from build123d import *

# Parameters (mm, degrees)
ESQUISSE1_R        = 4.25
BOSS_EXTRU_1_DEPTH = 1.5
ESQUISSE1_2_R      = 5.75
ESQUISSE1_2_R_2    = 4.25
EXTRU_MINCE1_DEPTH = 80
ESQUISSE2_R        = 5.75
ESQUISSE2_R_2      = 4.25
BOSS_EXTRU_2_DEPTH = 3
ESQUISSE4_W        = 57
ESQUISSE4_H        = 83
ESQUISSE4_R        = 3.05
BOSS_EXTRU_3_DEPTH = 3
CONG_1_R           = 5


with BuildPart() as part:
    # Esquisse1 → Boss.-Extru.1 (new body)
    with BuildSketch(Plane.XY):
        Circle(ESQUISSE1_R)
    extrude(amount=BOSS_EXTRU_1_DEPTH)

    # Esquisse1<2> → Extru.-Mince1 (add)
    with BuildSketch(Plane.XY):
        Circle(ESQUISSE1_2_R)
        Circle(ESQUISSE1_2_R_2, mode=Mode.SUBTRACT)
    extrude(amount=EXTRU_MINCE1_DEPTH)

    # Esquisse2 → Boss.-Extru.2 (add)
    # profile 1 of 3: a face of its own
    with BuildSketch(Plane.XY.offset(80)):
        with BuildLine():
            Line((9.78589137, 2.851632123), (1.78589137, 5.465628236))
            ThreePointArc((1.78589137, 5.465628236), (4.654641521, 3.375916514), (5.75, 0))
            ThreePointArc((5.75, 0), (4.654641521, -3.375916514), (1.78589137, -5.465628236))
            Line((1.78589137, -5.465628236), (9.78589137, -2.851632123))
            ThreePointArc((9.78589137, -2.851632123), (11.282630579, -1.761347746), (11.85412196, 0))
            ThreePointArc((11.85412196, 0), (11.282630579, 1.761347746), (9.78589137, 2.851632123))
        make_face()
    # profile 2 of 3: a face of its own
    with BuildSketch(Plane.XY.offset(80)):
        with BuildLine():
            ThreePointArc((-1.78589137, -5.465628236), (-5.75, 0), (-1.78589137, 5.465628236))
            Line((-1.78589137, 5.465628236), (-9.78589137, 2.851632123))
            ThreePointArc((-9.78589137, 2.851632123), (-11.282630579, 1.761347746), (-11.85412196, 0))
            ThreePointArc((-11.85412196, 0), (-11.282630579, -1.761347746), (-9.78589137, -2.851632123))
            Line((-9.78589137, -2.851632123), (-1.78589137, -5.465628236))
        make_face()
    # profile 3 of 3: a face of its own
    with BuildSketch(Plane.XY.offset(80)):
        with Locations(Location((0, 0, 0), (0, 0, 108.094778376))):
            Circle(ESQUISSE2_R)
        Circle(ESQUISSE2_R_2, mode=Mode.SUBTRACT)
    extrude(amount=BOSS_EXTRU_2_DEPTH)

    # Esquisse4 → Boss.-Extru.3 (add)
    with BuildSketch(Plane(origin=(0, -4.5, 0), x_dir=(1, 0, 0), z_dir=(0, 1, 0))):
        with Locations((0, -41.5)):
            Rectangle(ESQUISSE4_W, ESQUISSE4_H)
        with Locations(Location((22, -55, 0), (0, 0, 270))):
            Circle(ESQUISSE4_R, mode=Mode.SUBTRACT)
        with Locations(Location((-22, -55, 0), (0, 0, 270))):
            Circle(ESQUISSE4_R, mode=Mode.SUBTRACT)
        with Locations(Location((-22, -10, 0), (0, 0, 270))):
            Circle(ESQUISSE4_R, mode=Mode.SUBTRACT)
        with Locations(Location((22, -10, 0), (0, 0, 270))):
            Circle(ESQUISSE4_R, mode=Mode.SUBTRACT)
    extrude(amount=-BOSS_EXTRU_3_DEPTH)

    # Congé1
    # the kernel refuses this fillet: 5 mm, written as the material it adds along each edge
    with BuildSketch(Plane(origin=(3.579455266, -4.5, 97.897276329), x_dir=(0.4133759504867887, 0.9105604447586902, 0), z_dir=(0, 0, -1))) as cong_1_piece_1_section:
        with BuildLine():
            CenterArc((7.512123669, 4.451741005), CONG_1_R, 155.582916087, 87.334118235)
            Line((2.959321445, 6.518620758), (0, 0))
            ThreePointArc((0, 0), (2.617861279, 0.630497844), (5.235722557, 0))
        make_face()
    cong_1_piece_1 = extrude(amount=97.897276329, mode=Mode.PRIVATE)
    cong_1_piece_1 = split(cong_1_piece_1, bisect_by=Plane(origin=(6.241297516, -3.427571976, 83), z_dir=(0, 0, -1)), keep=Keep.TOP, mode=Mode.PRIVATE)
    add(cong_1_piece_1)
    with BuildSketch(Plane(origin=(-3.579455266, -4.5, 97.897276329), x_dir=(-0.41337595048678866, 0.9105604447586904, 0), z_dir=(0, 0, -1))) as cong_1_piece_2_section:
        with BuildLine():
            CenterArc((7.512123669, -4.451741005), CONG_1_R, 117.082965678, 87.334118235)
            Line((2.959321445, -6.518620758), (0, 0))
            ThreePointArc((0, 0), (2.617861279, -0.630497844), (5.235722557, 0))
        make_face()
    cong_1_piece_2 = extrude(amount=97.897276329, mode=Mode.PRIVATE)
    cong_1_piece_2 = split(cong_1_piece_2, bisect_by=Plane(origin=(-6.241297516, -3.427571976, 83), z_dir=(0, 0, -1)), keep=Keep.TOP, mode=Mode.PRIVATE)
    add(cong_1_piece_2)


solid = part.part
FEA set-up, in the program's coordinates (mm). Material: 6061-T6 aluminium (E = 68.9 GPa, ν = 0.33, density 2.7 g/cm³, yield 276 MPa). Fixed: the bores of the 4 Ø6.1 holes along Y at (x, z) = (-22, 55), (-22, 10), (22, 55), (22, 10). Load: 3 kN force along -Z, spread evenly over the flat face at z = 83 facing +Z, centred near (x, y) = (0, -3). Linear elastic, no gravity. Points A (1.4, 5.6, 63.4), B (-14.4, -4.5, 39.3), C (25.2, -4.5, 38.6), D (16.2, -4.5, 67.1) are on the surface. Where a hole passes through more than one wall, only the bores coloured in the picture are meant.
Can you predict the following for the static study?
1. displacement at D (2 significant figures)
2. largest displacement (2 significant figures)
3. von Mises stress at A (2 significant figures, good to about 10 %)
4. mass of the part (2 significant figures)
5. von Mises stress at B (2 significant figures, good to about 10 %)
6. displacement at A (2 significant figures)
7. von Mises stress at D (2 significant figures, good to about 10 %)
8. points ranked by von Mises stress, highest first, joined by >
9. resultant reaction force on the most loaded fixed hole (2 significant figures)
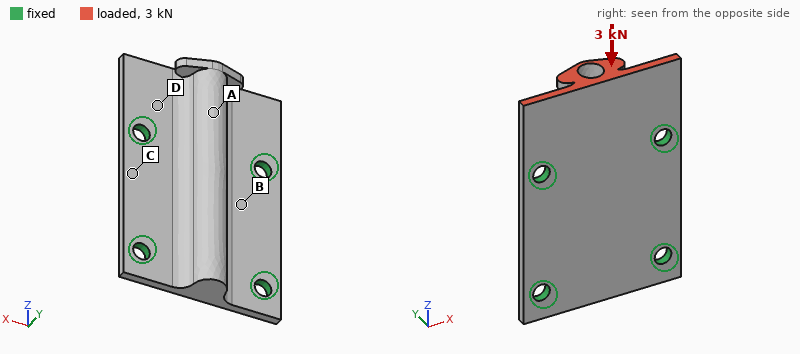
13 µm
59 µm
33 MPa
51 g
9.7 MPa
22 µm
19 MPa
A > D > B > C
1.1 kN
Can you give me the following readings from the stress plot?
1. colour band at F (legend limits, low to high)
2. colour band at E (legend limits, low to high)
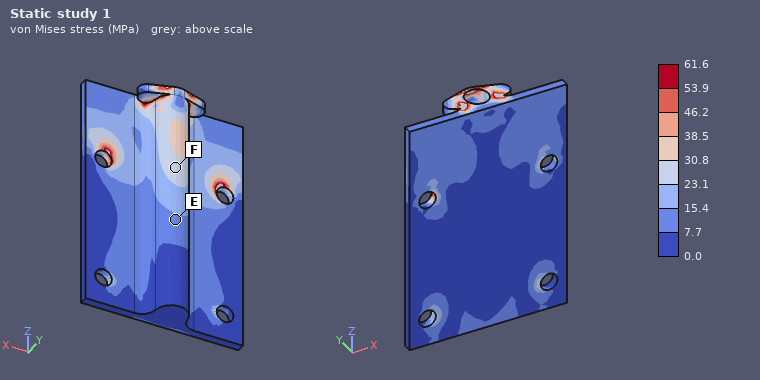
23.1 to 30.8 MPa
7.7 to 15.4 MPa
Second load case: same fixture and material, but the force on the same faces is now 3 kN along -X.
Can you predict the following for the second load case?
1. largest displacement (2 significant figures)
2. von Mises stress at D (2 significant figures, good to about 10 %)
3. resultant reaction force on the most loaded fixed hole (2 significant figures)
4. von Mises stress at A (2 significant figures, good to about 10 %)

63 µm
48 MPa
2.3 kN
20 MPa
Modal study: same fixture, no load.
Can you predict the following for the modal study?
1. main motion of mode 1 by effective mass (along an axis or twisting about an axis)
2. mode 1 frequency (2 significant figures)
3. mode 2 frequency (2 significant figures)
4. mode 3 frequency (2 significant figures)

along Y
4100 Hz
7000 Hz
7000 Hz
